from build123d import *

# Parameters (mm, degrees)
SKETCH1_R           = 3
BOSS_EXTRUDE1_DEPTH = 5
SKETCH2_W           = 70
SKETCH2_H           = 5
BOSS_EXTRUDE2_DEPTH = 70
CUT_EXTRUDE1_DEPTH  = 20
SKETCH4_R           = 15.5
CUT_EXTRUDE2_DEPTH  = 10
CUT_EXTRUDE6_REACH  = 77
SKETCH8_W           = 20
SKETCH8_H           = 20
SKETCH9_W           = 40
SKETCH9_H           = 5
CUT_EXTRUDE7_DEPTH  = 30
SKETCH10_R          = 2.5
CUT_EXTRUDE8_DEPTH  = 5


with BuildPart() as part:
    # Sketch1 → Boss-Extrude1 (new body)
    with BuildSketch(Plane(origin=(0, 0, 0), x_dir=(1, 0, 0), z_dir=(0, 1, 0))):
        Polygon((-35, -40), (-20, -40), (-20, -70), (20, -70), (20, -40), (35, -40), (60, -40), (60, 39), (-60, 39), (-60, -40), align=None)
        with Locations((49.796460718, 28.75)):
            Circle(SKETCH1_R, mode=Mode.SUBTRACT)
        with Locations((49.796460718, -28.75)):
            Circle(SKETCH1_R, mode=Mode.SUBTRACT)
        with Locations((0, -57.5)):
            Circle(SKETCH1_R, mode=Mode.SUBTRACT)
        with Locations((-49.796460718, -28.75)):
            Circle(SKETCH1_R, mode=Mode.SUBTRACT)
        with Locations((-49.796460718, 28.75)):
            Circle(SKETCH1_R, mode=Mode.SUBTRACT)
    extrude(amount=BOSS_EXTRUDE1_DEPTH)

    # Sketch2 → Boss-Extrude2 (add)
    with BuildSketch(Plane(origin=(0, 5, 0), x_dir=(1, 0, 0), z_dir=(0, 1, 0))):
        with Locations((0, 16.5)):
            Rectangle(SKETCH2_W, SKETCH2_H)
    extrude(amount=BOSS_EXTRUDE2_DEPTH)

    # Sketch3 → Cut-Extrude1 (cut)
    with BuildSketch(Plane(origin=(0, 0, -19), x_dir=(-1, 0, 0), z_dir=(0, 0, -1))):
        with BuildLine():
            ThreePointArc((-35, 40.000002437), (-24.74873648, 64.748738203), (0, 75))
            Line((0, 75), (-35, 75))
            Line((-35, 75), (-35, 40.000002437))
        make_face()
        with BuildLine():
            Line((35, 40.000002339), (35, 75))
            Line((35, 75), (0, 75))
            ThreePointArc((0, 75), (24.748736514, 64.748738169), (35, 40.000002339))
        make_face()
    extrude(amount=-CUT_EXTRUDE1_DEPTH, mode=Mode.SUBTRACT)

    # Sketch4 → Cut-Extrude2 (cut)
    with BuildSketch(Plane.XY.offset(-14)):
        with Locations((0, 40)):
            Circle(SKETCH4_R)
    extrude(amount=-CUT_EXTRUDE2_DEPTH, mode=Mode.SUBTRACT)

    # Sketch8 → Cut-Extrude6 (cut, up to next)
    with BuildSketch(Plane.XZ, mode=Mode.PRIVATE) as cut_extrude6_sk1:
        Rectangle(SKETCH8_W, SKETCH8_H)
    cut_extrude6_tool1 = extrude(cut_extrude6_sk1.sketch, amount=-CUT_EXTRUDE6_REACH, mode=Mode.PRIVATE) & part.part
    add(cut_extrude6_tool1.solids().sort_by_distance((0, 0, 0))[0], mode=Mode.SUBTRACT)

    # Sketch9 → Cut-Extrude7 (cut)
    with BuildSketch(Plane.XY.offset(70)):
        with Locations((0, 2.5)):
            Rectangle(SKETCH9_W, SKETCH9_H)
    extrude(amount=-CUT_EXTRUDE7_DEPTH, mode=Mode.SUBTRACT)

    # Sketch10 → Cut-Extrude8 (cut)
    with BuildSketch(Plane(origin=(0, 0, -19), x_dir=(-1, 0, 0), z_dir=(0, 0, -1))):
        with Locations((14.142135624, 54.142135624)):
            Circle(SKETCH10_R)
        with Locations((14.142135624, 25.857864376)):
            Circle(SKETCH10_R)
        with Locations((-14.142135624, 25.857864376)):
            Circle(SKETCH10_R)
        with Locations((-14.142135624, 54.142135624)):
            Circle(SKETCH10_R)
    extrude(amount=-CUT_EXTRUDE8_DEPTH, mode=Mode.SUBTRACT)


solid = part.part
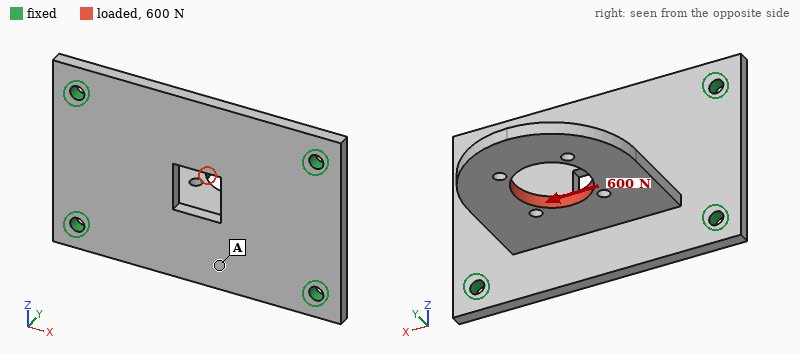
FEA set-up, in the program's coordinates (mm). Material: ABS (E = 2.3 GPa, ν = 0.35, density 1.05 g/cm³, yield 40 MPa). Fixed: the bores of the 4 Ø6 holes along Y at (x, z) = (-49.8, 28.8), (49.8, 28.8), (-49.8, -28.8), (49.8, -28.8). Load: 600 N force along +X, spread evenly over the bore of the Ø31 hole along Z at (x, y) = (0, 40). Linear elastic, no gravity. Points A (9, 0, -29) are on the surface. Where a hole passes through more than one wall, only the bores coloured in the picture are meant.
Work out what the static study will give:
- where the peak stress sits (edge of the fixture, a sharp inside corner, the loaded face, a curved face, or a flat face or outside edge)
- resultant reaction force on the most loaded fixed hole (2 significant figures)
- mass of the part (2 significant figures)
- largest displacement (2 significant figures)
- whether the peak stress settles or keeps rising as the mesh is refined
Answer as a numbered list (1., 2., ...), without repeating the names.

1. edge of the fixture
2. 330 N
3. 66 g
4. 0.97 mm
5. keeps rising
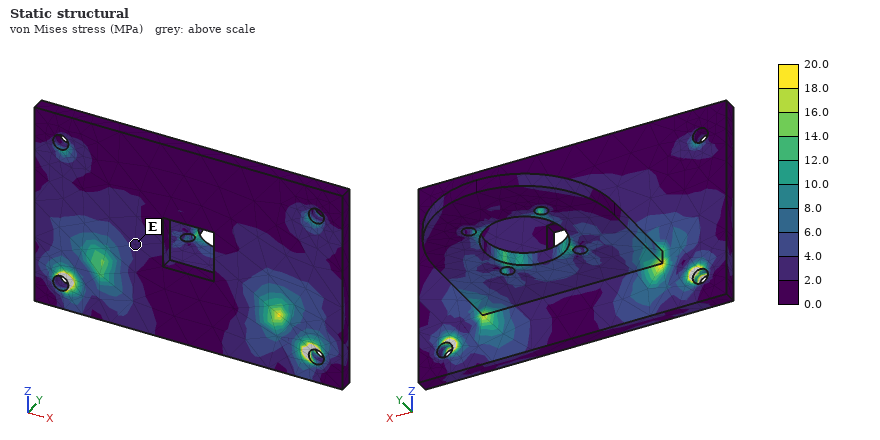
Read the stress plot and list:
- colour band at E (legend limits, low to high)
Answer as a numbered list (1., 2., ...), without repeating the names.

1. 2.0 to 4.0 MPa
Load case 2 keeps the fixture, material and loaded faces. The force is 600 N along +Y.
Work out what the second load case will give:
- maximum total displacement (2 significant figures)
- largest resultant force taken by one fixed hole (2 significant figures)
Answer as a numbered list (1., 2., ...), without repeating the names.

1. 0.64 mm
2. 270 N
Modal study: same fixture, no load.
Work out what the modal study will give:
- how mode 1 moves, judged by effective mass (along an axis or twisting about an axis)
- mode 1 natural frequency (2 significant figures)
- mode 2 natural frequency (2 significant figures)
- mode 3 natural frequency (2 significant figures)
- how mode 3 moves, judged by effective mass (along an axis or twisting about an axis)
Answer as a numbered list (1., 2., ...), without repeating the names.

1. along Z
2. 230 Hz
3. 650 Hz
4. 820 Hz
5. along Y
